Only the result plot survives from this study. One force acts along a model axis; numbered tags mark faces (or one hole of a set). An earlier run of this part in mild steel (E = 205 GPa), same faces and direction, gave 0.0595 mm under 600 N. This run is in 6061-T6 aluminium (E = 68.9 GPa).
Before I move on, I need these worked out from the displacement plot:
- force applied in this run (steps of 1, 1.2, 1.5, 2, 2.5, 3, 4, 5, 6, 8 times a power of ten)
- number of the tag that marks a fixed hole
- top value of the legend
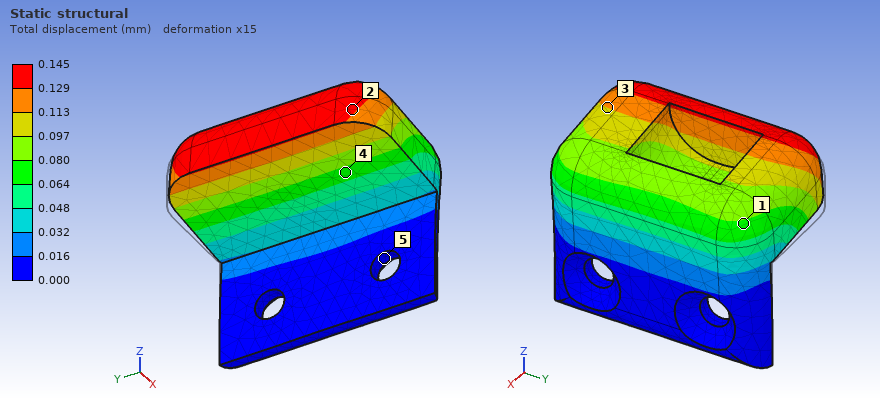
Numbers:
500 N
5
0.145 mm
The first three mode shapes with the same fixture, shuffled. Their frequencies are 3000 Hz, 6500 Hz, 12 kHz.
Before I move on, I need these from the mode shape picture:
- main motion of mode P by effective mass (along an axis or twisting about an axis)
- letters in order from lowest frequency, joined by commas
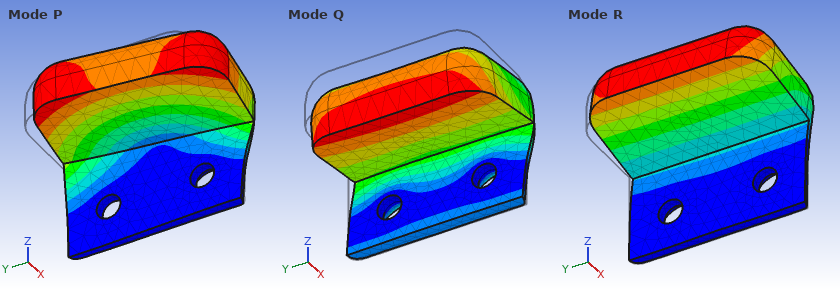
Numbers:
along Y
R, P, Q
